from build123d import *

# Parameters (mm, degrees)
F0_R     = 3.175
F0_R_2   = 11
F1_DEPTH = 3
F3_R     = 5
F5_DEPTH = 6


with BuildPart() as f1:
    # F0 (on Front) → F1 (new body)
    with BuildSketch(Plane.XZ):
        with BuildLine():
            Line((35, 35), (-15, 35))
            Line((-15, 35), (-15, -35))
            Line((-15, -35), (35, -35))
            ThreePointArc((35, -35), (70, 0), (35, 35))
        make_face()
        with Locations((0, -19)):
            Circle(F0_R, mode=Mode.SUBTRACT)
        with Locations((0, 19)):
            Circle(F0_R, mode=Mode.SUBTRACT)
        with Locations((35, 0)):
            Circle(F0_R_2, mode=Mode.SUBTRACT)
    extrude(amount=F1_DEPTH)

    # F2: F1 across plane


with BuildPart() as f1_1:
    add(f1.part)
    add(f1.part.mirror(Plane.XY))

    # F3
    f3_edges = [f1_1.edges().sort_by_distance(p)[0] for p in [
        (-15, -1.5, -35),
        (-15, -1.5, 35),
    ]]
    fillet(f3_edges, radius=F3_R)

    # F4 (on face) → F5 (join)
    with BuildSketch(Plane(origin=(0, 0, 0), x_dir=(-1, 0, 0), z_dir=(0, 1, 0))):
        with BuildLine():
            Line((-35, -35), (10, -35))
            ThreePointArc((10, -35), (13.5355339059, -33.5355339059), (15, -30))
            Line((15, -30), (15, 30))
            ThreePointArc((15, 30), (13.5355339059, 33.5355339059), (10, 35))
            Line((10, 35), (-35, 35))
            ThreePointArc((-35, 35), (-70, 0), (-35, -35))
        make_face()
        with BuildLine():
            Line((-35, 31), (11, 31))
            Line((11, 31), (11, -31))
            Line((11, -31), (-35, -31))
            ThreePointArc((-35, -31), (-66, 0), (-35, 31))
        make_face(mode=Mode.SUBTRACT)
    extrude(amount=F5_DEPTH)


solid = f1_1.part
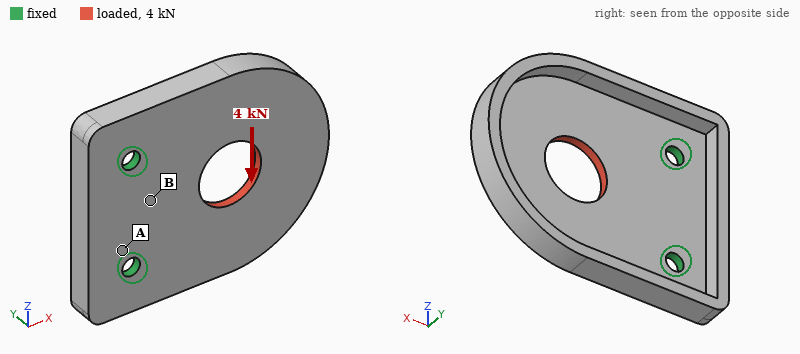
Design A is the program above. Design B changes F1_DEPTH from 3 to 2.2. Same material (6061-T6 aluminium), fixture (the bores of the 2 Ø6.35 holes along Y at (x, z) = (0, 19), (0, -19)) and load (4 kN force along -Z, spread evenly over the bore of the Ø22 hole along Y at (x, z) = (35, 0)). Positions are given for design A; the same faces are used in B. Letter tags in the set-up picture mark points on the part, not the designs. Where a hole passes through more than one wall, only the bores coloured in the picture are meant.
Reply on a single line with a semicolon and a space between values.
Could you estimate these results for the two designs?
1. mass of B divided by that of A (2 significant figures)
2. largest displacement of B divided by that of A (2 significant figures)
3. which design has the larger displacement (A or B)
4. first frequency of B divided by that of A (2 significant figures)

0.81; 1.4; B; 0.79
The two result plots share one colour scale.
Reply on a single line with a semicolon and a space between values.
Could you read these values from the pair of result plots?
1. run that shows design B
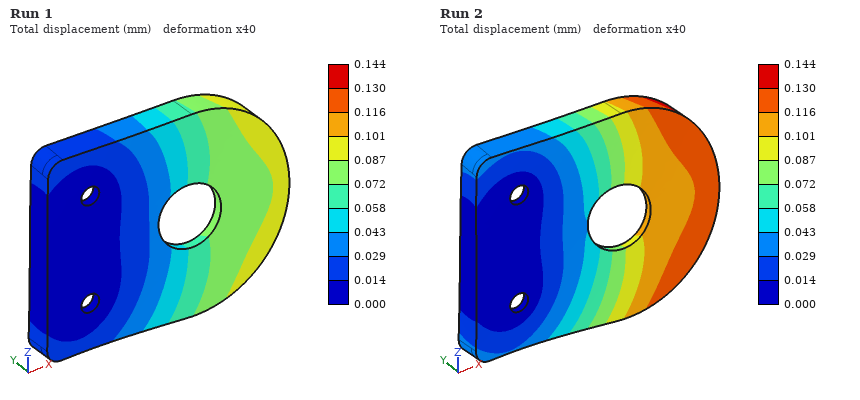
Run 2
